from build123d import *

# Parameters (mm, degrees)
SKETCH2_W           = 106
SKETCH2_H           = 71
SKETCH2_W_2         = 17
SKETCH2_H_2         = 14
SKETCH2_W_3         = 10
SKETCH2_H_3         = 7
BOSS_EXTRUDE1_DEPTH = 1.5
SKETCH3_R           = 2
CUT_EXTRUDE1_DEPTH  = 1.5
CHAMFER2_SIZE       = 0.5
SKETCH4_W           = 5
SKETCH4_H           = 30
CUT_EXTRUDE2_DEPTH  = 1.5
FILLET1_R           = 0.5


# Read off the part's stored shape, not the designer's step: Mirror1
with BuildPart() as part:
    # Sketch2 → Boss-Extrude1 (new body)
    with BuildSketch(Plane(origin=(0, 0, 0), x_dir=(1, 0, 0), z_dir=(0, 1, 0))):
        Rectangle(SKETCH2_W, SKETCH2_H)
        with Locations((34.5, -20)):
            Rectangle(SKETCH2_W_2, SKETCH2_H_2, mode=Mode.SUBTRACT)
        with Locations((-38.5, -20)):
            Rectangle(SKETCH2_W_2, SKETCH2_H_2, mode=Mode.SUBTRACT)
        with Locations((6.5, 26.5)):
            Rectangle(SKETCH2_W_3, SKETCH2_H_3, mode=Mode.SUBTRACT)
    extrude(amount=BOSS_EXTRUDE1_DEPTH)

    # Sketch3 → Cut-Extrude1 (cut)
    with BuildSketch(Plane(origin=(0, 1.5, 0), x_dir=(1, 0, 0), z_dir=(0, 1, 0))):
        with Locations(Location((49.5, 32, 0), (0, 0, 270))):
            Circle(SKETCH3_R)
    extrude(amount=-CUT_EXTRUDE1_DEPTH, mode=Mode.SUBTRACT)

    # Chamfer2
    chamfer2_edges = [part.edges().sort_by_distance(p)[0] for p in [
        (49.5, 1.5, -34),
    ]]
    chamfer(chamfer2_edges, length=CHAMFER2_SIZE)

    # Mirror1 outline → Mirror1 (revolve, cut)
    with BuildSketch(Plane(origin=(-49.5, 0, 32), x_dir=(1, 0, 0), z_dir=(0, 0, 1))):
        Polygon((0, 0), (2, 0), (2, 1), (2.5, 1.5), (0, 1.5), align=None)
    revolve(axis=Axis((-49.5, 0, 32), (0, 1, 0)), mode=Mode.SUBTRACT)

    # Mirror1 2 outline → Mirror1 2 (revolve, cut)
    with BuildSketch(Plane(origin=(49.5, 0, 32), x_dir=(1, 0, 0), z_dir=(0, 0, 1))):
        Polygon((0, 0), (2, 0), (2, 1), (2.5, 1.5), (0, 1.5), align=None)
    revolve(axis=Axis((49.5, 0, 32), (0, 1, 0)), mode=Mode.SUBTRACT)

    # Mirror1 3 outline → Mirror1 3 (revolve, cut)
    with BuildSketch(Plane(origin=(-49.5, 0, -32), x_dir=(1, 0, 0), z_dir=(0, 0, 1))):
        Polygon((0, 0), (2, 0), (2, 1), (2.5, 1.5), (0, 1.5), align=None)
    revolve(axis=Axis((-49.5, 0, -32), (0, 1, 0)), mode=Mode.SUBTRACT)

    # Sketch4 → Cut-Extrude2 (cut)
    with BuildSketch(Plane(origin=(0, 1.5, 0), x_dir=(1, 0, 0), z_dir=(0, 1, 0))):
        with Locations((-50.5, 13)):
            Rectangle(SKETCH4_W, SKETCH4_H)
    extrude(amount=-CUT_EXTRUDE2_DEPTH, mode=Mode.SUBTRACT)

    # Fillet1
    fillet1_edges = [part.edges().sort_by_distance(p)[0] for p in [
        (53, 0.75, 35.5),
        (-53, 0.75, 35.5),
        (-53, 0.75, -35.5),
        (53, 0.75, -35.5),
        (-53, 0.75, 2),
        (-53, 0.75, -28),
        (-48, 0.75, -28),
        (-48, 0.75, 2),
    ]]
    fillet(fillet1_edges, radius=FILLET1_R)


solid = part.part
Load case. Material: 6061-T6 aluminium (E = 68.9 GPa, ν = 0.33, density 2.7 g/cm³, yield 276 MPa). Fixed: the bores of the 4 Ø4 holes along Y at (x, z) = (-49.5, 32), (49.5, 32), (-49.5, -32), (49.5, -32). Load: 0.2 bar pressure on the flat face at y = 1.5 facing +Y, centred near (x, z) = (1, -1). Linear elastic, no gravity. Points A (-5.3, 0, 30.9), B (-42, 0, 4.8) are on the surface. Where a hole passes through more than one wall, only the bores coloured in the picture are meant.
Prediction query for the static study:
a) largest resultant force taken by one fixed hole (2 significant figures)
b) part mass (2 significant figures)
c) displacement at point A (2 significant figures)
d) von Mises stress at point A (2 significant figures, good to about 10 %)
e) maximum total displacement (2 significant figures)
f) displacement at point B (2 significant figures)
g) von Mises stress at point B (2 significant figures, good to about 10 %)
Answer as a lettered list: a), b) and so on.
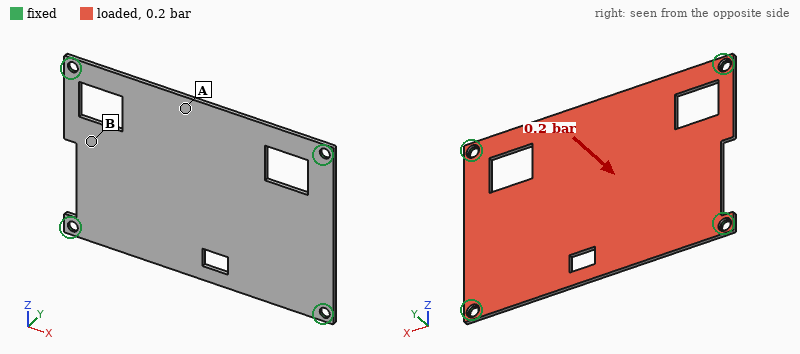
a) 40 N
b) 27 g
c) 0.43 mm
d) 30 MPa
e) 0.45 mm
f) 0.16 mm
g) 15 MPa
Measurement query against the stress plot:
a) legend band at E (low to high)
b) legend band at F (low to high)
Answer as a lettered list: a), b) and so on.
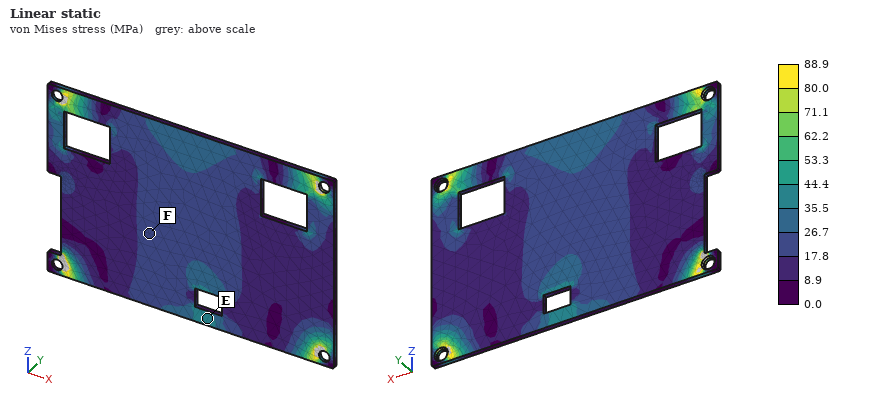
a) 35.5 to 44.4 MPa
b) 17.8 to 26.7 MPa
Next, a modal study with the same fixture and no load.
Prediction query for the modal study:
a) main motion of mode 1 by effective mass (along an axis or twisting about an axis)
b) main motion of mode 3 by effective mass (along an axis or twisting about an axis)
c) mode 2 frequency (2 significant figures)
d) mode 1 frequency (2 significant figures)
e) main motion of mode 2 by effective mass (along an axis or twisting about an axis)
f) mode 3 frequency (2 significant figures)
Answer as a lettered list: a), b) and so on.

a) along Y
b) twisting about Z
c) 1000 Hz
d) 600 Hz
e) twisting about X
f) 1500 Hz
